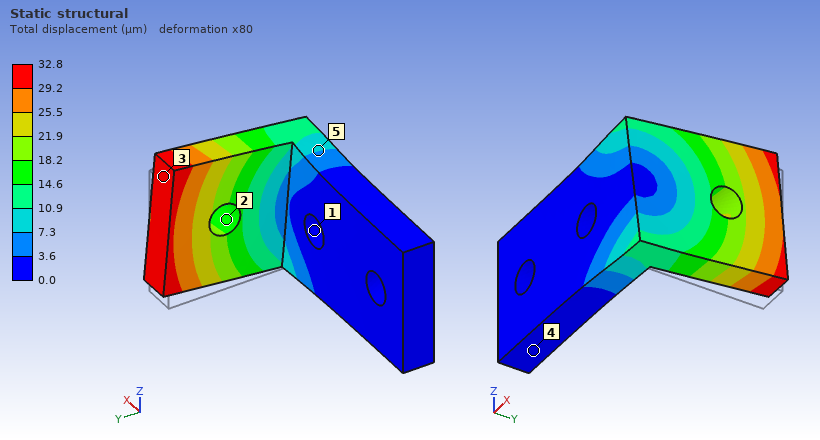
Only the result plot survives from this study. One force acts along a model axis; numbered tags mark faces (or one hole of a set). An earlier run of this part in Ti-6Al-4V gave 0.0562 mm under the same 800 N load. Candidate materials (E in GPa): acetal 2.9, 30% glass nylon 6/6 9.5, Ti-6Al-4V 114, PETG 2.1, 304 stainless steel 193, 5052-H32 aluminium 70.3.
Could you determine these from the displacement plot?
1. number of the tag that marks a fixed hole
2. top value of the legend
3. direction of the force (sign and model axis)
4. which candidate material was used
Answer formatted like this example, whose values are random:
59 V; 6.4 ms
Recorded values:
1; 32.8 µm; +Z; 304 stainless steel
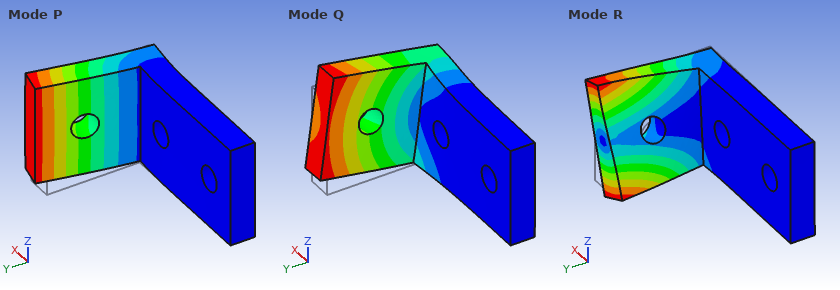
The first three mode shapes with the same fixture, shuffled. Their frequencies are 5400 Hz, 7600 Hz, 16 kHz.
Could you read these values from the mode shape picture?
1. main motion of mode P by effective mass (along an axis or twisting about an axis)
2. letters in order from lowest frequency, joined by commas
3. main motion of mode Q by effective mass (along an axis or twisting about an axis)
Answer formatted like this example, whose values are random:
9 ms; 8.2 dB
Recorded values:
along X; P, Q, R; along Z
